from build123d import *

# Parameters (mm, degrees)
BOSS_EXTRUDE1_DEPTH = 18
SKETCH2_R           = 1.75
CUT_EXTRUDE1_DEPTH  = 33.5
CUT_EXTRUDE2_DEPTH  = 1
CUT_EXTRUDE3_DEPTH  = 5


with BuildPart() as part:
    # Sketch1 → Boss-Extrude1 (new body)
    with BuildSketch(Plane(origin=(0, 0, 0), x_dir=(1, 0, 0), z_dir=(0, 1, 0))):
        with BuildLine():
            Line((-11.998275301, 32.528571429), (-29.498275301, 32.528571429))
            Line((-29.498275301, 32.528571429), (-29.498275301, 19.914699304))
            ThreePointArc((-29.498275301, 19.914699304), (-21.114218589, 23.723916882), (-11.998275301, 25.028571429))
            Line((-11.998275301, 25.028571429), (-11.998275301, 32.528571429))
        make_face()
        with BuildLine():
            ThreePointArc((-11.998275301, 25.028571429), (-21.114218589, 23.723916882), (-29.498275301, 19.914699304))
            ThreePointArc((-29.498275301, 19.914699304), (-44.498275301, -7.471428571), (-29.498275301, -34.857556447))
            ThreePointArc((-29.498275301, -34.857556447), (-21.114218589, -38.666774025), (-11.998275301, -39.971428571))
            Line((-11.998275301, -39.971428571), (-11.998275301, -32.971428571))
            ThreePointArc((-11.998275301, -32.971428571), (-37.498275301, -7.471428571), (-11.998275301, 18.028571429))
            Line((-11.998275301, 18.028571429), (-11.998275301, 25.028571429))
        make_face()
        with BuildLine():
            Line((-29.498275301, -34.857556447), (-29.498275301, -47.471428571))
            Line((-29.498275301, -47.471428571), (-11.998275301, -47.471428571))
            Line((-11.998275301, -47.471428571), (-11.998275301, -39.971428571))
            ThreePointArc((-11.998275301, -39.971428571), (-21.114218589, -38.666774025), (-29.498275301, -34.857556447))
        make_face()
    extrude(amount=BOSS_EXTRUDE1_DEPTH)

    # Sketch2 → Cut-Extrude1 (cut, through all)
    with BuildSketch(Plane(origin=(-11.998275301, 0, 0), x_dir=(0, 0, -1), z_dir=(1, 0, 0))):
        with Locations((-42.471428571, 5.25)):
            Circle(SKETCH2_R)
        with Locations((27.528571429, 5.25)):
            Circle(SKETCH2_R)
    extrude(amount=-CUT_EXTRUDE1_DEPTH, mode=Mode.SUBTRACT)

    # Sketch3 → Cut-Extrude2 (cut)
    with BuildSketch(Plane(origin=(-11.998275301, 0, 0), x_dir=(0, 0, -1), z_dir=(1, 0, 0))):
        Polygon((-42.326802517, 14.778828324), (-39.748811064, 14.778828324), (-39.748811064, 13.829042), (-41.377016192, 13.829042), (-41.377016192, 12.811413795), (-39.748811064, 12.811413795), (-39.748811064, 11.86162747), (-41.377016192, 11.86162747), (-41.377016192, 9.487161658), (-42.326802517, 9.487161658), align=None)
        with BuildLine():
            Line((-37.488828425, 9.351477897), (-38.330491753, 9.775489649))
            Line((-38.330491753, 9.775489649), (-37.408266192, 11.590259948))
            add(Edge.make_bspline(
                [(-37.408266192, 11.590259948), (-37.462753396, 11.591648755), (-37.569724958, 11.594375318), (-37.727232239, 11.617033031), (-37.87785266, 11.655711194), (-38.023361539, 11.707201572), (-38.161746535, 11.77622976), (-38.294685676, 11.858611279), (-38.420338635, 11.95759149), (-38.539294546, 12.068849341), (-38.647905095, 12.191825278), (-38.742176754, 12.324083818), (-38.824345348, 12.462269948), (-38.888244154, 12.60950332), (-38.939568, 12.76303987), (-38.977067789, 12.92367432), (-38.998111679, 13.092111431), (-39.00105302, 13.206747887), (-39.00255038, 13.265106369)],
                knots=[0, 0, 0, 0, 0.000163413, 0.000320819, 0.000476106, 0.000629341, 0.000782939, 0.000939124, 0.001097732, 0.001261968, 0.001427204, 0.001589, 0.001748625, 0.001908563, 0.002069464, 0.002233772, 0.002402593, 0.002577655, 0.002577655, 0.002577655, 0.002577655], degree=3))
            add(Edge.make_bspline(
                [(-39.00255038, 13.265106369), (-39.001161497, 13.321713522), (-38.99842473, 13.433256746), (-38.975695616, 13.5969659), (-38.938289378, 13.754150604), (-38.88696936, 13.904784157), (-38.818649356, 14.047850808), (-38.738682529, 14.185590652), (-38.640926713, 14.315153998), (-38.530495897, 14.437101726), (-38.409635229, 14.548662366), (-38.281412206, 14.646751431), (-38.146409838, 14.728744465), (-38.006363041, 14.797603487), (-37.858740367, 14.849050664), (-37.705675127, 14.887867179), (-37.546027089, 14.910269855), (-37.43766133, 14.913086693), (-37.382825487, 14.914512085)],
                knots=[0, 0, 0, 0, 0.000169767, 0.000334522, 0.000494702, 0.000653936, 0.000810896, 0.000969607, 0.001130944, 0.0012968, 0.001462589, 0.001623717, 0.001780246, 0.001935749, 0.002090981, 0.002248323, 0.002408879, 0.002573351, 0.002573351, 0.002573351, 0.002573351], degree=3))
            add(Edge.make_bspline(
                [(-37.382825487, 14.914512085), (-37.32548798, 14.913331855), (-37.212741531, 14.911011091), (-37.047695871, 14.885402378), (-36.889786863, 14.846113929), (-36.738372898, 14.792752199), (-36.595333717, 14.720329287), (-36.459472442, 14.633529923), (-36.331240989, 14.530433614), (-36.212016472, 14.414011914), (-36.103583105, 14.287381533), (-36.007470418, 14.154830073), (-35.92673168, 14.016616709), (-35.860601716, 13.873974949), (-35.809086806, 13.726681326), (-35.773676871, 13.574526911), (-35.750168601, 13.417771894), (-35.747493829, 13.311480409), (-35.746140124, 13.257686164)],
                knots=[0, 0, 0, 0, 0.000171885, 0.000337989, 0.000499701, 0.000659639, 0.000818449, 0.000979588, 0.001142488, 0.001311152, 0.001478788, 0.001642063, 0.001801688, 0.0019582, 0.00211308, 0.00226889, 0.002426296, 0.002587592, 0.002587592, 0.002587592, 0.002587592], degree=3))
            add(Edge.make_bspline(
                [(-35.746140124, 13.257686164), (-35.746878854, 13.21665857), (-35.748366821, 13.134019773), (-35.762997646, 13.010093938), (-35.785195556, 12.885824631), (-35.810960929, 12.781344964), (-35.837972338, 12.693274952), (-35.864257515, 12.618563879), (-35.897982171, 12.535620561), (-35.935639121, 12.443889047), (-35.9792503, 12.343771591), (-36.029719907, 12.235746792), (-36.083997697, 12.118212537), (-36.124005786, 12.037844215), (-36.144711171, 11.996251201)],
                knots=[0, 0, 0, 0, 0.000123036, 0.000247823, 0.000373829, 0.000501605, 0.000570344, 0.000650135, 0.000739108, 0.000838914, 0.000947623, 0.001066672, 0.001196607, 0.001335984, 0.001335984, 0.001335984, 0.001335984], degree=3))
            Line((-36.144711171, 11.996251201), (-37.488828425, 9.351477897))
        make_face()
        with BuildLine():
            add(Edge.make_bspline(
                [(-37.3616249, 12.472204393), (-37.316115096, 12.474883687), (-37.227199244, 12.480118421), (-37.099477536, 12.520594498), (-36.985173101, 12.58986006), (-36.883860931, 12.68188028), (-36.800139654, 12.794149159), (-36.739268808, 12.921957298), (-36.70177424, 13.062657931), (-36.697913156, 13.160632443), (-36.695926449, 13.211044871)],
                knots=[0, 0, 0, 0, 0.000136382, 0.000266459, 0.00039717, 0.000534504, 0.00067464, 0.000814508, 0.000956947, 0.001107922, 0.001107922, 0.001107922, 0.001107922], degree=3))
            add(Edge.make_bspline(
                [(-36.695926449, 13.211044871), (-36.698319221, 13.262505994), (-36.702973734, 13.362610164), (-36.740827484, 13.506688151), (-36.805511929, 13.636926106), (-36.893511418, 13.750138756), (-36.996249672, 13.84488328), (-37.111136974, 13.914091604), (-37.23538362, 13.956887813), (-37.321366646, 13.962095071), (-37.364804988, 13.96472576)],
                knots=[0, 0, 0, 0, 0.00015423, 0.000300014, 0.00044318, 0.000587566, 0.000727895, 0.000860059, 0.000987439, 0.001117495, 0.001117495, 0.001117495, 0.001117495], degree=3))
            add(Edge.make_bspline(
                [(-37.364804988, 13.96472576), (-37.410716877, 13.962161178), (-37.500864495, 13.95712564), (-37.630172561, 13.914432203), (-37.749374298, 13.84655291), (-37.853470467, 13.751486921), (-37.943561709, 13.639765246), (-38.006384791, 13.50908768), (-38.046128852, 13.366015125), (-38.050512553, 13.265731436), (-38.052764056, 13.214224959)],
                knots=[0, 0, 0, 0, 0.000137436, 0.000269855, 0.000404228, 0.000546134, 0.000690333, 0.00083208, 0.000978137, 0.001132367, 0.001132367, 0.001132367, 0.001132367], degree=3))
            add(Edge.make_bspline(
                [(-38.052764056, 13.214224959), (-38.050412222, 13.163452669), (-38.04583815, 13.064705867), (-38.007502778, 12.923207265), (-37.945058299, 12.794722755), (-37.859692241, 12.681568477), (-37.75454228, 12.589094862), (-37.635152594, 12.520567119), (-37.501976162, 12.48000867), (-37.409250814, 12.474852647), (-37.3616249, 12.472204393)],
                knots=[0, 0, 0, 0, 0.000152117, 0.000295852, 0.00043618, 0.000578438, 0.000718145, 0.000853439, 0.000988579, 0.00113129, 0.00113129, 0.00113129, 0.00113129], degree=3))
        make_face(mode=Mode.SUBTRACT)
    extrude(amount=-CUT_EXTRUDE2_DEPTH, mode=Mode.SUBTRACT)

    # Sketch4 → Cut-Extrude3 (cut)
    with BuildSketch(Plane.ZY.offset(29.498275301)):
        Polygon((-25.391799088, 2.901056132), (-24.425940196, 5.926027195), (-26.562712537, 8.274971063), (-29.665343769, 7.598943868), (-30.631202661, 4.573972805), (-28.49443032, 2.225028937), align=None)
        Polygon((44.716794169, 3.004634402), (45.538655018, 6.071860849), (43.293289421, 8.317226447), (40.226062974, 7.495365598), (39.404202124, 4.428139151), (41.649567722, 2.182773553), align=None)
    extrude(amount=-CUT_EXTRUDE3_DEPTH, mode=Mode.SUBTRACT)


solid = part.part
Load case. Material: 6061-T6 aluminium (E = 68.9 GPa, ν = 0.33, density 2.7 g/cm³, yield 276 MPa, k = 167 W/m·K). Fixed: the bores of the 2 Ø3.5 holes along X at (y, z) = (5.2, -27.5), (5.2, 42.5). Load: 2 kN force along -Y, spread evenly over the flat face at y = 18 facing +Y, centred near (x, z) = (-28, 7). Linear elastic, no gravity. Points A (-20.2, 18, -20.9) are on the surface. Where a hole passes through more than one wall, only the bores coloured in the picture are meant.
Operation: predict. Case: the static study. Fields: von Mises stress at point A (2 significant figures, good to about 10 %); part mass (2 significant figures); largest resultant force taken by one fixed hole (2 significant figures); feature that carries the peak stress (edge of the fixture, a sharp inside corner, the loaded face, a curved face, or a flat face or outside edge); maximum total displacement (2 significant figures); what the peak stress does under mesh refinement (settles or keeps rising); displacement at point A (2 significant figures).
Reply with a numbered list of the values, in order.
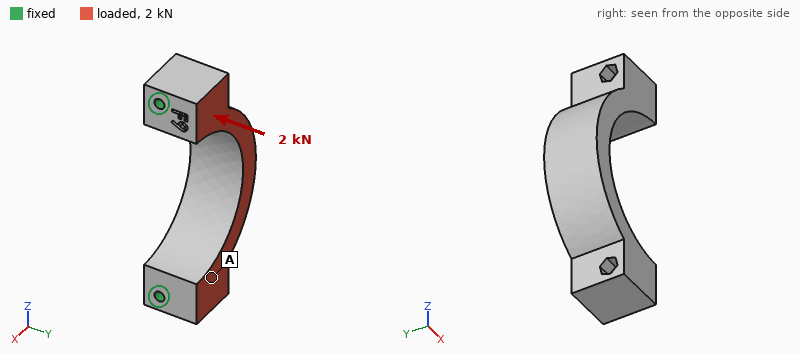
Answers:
1. 12 MPa
2. 45 g
3. 1.0 kN
4. edge of the fixture
5. 39 µm
6. keeps rising
7. 11 µm
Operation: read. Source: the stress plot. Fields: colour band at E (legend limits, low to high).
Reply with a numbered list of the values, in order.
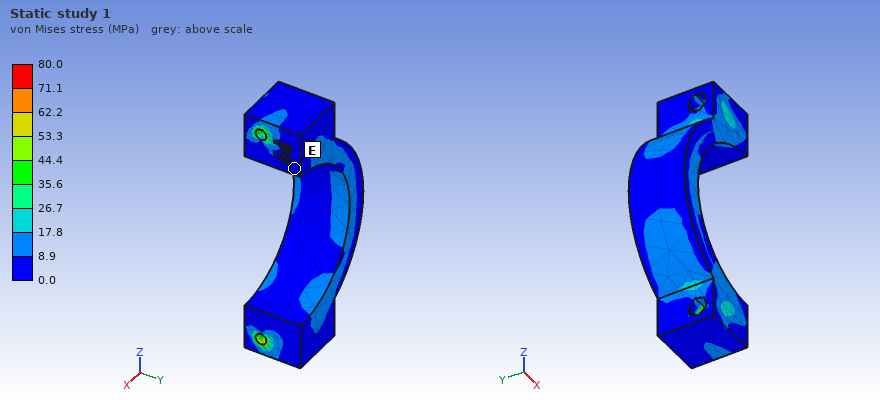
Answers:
1. 0.0 to 8.9 MPa
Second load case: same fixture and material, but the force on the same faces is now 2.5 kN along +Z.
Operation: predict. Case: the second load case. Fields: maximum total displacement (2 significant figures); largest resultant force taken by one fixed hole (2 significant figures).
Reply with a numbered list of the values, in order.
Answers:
1. 14 µm
2. 1.3 kN
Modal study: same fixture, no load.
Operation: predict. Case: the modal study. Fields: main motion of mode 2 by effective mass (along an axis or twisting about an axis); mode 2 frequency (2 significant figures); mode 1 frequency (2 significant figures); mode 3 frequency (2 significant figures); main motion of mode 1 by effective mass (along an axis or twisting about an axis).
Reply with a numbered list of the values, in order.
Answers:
1. along Z
2. 13 kHz
3. 6600 Hz
4. 17 kHz
5. along Y
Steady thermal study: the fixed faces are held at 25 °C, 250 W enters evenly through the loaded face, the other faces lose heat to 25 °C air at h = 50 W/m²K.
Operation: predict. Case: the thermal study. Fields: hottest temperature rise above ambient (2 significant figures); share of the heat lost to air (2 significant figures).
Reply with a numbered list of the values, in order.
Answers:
1. 81 K
2. 4.0 %
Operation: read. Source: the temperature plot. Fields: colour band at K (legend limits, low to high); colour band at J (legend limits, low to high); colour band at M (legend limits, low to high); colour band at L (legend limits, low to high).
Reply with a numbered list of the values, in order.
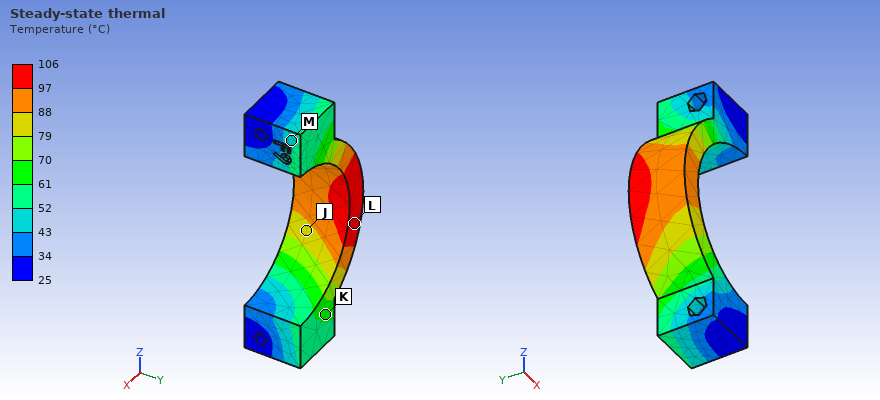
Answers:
1. 61 to 70 °C
2. 79 to 88 °C
3. 43 to 52 °C
4. 97 to 106 °C
